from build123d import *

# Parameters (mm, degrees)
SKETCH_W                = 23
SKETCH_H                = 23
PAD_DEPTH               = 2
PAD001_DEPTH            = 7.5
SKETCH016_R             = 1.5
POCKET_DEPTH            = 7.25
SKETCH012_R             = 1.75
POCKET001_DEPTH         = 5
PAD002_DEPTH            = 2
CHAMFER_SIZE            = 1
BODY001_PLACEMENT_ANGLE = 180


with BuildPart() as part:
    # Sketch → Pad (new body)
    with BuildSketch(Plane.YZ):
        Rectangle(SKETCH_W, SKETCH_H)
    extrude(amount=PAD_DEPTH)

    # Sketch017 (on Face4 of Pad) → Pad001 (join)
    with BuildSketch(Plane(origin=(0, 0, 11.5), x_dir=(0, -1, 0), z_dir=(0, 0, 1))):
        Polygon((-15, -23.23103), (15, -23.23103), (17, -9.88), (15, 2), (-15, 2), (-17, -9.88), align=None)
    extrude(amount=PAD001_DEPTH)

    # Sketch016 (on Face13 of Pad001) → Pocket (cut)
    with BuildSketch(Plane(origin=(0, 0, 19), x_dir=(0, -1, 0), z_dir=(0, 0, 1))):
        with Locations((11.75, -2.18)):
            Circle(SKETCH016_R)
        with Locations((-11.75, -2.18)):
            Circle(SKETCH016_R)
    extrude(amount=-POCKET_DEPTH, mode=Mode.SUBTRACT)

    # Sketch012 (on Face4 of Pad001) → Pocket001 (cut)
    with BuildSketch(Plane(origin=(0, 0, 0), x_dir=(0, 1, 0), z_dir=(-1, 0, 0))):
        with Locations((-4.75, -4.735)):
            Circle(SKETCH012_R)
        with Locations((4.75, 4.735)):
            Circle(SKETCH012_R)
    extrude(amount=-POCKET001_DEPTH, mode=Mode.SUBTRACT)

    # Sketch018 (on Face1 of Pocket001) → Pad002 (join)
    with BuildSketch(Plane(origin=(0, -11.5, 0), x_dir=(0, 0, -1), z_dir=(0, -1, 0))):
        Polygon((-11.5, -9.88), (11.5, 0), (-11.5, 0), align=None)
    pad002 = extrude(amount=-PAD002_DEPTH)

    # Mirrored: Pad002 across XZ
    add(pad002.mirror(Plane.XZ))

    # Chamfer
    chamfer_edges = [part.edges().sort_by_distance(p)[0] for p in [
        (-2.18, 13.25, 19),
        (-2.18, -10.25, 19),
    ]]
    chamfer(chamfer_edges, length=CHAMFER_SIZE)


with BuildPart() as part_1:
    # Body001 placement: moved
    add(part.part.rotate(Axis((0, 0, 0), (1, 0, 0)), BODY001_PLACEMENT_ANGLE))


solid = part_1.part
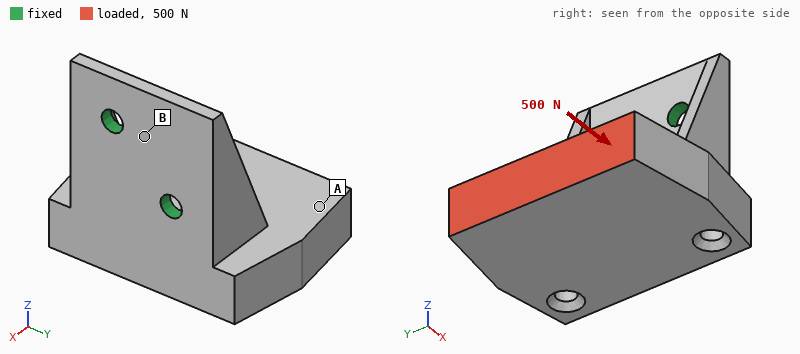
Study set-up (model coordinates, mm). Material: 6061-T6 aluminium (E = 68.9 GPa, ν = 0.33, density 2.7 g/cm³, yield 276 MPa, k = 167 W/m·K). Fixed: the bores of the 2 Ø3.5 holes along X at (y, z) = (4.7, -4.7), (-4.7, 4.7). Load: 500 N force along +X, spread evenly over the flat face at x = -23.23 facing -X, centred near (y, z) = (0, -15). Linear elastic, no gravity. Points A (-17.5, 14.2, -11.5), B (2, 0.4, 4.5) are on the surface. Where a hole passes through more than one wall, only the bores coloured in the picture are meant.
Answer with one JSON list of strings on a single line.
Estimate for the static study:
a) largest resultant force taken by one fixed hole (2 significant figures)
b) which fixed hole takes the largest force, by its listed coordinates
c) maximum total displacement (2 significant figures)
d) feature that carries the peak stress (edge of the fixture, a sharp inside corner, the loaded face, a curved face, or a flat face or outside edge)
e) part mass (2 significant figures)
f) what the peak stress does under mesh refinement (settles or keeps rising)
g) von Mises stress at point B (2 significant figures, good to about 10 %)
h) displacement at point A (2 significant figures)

["510 N", "(4.7, -4.7)", "0.25 mm", "edge of the fixture", "20 g", "keeps rising", "45 MPa", "0.14 mm"]
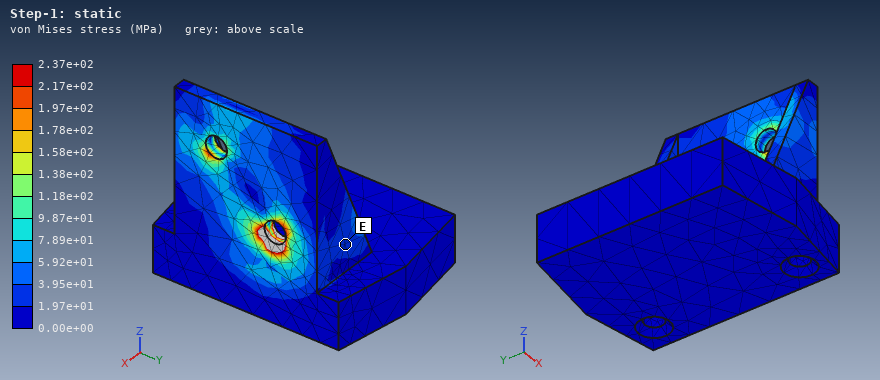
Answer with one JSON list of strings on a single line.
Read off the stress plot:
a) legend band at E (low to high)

["1.97e+01 to 3.95e+01 MPa"]
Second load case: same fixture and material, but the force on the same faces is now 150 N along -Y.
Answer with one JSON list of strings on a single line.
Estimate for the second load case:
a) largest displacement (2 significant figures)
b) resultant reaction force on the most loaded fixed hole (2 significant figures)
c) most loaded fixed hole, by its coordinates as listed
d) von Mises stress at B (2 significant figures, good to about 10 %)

["0.12 mm", "260 N", "(4.7, -4.7)", "13 MPa"]
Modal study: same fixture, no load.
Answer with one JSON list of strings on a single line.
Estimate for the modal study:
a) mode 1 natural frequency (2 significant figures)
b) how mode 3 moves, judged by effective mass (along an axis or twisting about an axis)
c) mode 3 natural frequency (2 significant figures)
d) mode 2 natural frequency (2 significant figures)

["1800 Hz", "along X", "8500 Hz", "3200 Hz"]
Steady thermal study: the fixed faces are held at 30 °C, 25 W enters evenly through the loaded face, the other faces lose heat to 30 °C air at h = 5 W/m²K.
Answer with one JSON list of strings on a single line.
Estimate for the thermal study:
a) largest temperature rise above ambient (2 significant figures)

["39 K"]
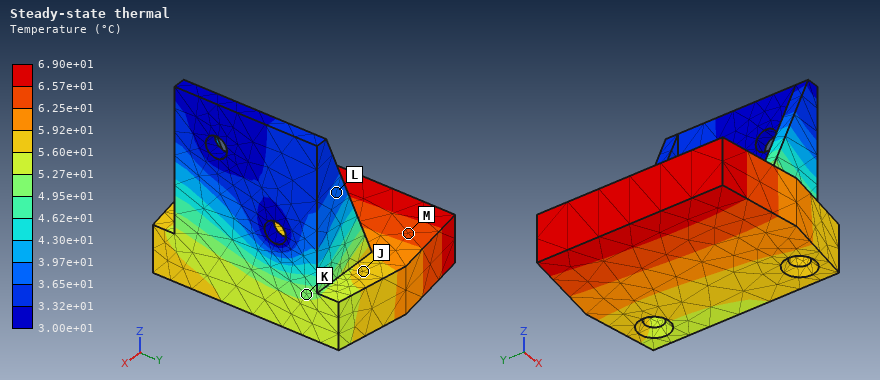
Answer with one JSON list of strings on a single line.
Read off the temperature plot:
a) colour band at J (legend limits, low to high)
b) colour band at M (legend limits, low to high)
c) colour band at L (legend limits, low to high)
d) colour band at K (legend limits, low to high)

["5.60e+01 to 5.92e+01 °C", "6.25e+01 to 6.57e+01 °C", "3.65e+01 to 3.97e+01 °C", "4.95e+01 to 5.27e+01 °C"]
